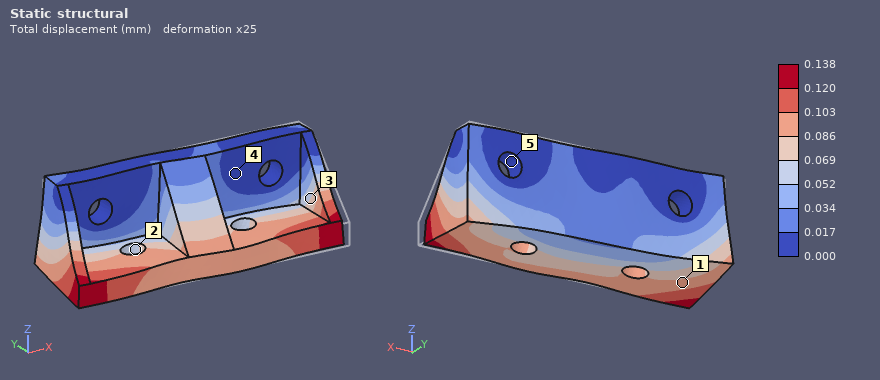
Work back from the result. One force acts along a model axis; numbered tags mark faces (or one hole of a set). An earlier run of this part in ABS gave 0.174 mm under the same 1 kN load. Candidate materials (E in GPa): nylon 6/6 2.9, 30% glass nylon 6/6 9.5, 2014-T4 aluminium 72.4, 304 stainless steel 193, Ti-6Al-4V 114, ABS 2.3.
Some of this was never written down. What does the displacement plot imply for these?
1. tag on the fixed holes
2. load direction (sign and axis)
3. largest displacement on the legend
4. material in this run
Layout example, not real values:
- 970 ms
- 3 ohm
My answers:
- 5
- -X
- 0.138 mm
- nylon 6/6
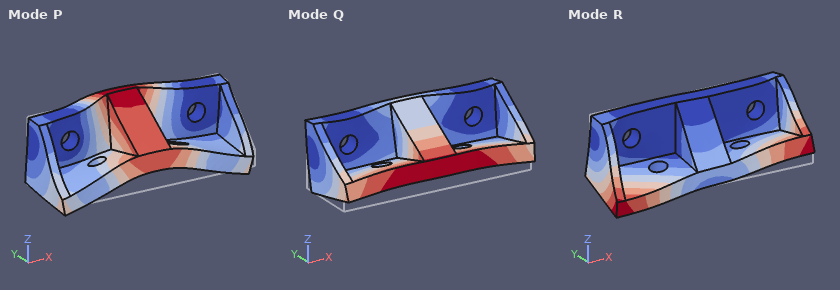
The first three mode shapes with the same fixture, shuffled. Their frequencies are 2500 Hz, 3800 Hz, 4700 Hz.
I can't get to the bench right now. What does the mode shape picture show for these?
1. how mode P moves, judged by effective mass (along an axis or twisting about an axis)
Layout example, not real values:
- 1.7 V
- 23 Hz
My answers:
- along Y
